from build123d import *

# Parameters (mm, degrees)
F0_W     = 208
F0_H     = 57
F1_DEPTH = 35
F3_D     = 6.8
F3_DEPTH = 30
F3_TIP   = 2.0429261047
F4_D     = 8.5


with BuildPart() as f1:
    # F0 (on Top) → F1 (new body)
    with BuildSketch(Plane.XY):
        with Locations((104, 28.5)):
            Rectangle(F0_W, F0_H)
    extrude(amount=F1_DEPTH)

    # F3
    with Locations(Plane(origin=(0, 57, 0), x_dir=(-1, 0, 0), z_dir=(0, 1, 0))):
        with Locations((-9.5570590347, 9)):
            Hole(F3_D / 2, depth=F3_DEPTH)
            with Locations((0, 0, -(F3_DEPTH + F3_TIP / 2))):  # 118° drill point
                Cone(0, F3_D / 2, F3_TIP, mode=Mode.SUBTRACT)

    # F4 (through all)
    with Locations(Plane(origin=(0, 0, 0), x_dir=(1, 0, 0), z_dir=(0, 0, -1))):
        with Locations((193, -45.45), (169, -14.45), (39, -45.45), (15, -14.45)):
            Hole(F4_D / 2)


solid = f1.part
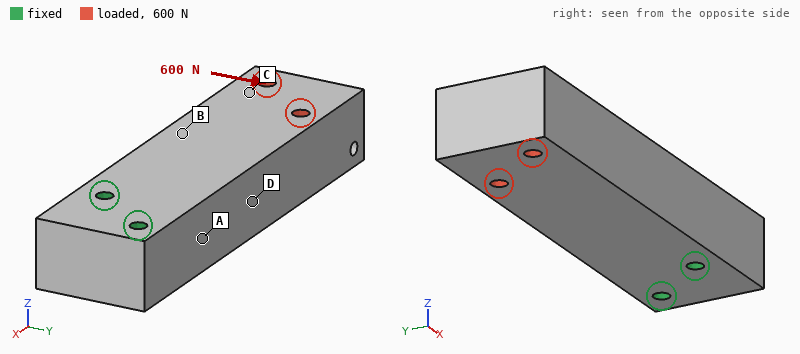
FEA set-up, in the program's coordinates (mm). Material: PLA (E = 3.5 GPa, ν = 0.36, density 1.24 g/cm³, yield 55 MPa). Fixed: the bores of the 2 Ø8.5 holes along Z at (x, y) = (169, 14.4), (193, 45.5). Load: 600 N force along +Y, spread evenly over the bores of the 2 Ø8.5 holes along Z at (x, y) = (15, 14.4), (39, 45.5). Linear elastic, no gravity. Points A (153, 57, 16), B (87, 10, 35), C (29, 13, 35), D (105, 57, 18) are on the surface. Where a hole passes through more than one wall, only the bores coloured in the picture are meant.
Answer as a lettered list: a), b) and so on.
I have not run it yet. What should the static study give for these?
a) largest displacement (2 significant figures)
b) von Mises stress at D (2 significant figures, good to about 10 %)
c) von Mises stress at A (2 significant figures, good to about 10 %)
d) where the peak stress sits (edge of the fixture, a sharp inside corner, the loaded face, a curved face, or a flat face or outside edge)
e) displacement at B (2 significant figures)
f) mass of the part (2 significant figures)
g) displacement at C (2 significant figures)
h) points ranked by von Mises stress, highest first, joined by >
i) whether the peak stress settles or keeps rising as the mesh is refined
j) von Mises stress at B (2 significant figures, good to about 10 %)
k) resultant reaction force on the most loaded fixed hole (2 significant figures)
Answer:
a) 0.55 mm
b) 2.5 MPa
c) 4.1 MPa
d) edge of the fixture
e) 0.20 mm
f) 500 g
g) 0.42 mm
h) A > D > B > C
i) keeps rising
j) 1.3 MPa
k) 2.3 kN
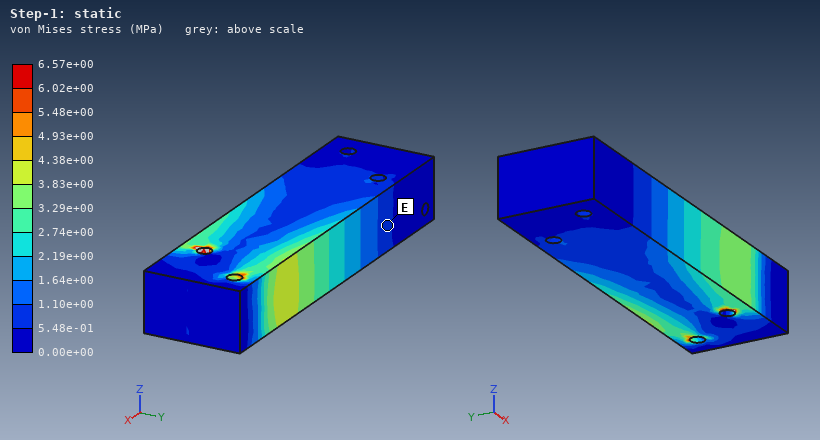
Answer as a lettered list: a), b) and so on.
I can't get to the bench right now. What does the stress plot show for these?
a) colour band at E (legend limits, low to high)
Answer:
a) 5.48e-01 to 1.10e+00 MPa
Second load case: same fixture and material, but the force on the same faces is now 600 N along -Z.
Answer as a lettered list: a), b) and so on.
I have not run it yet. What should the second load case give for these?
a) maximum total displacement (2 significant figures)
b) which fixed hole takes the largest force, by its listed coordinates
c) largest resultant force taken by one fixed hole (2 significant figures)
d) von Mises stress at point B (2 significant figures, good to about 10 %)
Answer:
a) 1.2 mm
b) (169, 14.4)
c) 980 N
d) 3.1 MPa
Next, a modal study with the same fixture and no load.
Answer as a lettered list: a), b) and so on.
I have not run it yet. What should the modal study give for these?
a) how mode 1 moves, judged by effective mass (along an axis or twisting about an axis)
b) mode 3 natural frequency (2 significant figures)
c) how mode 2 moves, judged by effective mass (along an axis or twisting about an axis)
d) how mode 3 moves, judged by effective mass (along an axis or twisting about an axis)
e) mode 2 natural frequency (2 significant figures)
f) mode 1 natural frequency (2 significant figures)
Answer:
a) along Z
b) 1200 Hz
c) along Y
d) twisting about X
e) 450 Hz
f) 310 Hz
